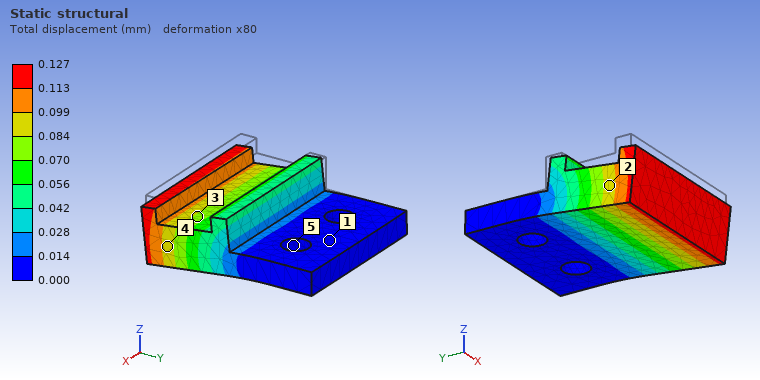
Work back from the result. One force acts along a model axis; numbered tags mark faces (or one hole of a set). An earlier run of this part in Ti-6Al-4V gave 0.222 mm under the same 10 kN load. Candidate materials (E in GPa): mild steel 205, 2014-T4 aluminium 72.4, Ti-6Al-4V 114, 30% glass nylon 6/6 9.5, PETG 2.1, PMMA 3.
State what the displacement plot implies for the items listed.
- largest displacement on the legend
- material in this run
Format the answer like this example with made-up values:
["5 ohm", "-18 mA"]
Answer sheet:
["0.127 mm", "mild steel"]
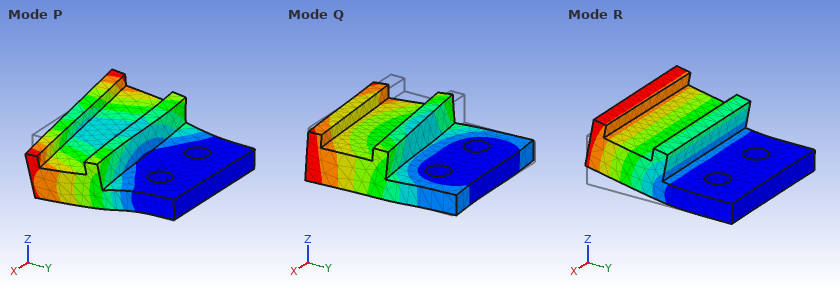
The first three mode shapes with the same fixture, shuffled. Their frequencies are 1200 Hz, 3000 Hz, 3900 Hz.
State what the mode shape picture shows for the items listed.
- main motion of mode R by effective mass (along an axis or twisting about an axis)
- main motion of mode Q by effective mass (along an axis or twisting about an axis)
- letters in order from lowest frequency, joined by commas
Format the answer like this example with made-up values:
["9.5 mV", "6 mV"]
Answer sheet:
["along Z", "along X", "R, P, Q"]
